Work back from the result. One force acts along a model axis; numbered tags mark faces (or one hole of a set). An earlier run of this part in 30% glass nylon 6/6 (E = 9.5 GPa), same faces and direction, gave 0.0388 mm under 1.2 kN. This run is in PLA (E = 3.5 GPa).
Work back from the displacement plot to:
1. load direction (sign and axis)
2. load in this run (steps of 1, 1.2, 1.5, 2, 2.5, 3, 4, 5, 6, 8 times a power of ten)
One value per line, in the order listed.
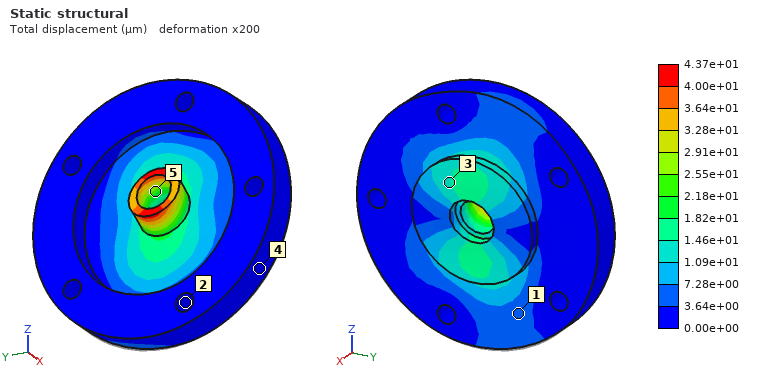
+Z
500 N
